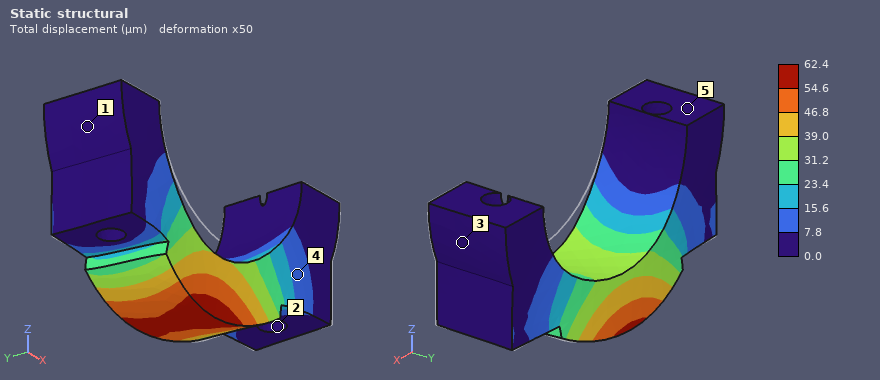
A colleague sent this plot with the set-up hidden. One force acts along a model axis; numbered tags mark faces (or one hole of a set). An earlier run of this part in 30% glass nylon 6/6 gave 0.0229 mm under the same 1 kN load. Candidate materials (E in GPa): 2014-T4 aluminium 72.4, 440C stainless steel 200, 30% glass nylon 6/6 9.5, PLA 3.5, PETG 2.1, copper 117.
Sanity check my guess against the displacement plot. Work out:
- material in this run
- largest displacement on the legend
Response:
PLA
62.4 µm
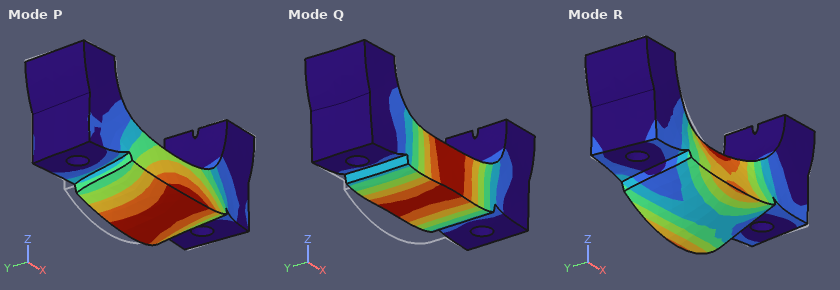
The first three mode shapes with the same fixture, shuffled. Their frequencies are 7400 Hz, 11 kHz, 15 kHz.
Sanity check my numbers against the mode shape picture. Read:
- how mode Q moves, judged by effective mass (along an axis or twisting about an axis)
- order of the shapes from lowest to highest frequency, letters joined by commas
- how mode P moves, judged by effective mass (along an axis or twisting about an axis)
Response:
along Z
P, Q, R
along Y
